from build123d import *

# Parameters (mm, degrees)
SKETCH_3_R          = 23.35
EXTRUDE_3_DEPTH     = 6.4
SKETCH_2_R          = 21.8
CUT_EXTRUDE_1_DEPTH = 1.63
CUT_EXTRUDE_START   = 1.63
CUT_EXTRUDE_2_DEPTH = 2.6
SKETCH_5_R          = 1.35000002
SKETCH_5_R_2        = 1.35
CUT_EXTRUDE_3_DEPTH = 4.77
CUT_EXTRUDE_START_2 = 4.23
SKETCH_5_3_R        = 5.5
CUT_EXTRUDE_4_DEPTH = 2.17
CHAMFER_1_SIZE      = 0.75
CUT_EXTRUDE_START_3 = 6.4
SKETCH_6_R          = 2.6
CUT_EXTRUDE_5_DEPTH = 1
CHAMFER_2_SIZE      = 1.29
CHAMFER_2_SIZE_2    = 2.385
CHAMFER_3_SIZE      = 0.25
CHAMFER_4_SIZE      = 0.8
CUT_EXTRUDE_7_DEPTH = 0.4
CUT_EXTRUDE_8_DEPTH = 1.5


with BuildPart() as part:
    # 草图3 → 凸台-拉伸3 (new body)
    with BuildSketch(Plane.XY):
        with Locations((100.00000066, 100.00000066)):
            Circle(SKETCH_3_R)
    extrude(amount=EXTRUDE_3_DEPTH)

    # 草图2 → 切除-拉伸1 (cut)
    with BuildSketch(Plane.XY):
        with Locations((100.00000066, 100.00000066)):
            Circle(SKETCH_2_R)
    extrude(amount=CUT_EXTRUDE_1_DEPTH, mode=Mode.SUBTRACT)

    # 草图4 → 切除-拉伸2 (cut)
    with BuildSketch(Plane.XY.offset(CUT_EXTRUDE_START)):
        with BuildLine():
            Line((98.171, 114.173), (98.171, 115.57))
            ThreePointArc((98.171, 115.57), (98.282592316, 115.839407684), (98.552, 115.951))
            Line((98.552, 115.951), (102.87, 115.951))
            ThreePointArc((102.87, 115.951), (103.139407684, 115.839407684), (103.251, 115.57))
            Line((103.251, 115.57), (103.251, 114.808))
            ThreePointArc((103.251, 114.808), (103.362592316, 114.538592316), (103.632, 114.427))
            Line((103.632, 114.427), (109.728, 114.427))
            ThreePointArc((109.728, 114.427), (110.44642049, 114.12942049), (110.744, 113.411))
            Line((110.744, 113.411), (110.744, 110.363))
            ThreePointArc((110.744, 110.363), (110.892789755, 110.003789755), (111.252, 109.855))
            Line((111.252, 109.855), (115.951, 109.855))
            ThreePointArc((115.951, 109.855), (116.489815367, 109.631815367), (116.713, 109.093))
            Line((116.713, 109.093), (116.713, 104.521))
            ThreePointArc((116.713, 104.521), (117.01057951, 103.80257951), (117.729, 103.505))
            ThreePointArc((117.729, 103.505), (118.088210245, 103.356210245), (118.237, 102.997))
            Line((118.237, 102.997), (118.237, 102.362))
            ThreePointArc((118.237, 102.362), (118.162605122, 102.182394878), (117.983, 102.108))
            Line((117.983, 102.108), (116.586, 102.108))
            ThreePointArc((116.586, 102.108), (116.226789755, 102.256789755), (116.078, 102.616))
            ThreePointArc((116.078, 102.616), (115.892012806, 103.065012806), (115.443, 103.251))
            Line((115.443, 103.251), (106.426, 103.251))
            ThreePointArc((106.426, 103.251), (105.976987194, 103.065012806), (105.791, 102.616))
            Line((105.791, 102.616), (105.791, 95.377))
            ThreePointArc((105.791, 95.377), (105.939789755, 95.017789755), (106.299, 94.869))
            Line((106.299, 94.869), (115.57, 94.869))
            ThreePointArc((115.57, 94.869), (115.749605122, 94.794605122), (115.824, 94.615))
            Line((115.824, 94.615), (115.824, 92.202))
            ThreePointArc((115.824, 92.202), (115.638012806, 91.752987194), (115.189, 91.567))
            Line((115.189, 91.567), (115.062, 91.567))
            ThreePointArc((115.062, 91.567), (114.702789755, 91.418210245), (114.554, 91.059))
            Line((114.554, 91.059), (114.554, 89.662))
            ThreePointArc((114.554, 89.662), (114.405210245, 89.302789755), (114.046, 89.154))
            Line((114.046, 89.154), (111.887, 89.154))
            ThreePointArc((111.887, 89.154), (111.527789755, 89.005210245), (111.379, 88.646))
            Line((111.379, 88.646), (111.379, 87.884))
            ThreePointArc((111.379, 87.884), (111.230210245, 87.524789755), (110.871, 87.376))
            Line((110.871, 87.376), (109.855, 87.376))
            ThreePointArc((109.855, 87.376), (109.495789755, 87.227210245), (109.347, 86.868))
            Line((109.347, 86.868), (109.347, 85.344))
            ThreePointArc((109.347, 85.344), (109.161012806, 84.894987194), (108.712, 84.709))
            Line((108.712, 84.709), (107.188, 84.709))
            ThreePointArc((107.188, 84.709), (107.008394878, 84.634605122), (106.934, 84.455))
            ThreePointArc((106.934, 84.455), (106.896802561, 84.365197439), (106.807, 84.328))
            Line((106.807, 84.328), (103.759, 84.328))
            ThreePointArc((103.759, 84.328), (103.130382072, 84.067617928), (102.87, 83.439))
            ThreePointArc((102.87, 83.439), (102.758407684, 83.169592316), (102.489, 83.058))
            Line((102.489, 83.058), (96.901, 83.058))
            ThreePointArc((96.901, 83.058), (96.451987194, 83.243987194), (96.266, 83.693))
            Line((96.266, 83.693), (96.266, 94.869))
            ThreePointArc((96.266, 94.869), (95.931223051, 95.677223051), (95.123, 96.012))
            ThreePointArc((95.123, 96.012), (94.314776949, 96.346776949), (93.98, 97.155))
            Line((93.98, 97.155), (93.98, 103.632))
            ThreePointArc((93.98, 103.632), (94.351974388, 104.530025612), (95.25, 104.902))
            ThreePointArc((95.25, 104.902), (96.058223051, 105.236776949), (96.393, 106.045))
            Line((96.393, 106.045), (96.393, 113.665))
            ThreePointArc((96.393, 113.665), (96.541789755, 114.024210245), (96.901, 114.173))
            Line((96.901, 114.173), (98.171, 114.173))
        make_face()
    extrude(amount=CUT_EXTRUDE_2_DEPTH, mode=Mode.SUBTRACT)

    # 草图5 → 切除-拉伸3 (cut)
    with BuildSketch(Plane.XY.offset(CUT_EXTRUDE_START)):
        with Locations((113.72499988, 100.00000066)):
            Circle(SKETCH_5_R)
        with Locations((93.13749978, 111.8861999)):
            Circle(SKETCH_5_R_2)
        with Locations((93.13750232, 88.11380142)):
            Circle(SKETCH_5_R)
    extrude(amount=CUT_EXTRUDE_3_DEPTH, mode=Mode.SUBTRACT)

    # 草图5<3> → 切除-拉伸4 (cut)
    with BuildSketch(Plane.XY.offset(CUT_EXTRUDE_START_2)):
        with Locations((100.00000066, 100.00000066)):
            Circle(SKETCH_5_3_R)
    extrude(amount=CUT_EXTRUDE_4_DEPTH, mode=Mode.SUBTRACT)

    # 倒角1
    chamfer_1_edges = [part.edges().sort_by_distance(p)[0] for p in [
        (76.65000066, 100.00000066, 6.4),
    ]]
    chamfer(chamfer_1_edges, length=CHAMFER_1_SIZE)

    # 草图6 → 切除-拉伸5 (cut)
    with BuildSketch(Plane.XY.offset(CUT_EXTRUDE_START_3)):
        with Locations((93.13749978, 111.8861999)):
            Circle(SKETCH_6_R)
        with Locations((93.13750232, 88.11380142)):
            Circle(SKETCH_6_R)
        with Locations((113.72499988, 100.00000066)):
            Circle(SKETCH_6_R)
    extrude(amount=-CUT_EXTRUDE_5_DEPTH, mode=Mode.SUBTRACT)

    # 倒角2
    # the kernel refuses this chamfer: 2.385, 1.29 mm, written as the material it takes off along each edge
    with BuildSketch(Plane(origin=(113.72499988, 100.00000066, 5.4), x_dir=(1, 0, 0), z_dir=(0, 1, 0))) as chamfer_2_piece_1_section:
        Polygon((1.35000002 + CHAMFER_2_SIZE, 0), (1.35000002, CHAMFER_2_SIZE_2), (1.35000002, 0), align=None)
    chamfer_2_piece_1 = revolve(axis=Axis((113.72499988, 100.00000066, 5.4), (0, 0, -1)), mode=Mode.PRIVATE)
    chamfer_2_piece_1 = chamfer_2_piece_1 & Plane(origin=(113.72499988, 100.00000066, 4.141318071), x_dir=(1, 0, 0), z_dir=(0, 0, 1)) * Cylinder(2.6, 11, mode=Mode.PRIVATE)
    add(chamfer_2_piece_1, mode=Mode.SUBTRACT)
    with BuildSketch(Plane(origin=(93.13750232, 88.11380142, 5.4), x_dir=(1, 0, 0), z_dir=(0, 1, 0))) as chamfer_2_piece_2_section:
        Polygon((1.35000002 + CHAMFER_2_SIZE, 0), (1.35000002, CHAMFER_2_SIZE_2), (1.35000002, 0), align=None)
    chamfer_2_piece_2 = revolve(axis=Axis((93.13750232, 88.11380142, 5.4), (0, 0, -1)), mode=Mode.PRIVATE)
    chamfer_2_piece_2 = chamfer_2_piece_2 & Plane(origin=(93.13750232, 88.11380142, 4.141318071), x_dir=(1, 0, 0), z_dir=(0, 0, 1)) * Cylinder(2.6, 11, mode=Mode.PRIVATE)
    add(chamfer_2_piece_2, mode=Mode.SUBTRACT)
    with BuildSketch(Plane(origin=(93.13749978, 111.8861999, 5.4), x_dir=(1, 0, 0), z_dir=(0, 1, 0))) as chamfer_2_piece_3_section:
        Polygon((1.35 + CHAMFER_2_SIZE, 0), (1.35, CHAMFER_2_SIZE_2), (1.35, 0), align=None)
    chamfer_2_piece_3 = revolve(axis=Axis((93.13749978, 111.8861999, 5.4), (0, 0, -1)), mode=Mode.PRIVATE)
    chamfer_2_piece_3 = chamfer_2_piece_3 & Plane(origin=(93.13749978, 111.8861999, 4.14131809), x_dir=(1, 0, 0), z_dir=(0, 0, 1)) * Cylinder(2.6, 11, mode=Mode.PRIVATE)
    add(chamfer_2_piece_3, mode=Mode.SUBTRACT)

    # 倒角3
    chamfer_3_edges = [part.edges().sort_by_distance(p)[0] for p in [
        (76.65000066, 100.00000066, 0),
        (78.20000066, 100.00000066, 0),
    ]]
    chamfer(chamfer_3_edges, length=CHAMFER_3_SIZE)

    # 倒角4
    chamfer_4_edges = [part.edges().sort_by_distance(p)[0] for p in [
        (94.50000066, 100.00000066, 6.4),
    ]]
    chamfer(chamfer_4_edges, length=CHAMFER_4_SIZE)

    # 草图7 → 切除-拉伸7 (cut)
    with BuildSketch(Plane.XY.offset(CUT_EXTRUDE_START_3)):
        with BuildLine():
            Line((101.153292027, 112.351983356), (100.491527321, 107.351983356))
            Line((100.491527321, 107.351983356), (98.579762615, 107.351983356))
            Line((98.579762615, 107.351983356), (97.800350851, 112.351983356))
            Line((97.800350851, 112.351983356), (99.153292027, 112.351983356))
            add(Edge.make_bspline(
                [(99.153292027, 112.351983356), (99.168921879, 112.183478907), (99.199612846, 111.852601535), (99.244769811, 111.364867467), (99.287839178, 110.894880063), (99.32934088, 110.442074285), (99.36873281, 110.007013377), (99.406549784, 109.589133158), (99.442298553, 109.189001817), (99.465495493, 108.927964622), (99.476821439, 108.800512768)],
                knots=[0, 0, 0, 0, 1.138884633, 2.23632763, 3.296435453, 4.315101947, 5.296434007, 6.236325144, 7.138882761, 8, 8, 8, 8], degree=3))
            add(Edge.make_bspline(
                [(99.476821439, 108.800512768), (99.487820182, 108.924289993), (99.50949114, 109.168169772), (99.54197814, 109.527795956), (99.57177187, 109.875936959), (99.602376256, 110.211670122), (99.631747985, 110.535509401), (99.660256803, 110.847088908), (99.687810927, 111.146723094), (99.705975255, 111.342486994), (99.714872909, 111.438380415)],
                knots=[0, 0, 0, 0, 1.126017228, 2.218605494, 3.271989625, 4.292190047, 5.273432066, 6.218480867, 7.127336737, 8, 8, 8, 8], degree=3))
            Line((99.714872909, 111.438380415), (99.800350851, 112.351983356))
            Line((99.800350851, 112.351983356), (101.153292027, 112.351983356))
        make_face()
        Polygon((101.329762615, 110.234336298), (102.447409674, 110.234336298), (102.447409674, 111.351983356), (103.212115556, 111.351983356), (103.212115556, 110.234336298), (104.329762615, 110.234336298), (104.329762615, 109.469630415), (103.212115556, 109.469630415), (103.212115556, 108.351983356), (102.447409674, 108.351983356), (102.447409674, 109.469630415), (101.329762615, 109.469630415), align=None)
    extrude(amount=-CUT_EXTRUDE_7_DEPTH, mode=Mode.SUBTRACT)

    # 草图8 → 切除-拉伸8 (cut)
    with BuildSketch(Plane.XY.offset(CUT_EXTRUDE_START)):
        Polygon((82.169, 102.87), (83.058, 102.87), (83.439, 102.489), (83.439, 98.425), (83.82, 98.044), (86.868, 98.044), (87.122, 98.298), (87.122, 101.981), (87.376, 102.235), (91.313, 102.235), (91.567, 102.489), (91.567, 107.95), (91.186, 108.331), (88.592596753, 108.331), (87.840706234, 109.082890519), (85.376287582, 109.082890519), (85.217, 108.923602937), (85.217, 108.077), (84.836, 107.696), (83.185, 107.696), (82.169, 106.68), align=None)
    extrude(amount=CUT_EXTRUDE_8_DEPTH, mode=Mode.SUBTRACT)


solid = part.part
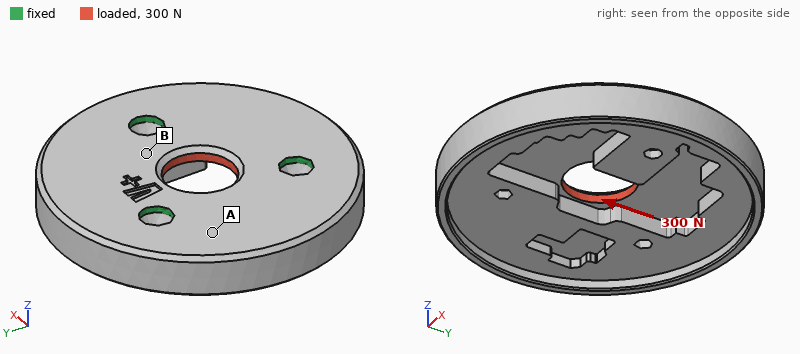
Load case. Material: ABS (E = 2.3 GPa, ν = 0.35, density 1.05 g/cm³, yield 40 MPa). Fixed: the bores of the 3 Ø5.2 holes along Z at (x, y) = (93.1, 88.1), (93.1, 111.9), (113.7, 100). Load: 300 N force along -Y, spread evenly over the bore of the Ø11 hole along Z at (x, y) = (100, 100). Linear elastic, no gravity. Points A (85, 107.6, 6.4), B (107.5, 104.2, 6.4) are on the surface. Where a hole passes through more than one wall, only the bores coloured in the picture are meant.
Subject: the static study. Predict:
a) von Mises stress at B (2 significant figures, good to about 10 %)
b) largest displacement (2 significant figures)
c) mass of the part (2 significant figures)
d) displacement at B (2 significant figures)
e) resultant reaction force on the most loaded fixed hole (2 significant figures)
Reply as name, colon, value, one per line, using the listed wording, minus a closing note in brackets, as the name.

von Mises stress at B: 2.4 MPa
largest displacement: 30 µm
mass of the part: 7.0 g
displacement at B: 13 µm
resultant reaction force on the most loaded fixed hole: 100 N
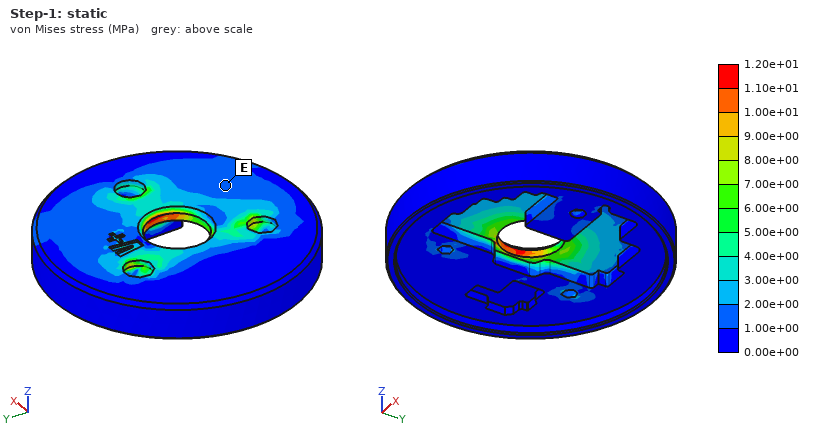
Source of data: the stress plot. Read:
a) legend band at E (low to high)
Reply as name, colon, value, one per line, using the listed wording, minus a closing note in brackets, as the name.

legend band at E: 1.00e+00 to 2.00e+00 MPa
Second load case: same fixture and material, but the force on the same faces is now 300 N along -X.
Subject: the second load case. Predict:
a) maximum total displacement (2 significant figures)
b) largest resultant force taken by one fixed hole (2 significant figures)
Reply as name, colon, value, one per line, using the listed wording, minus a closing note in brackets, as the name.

maximum total displacement: 23 µm
largest resultant force taken by one fixed hole: 100 N
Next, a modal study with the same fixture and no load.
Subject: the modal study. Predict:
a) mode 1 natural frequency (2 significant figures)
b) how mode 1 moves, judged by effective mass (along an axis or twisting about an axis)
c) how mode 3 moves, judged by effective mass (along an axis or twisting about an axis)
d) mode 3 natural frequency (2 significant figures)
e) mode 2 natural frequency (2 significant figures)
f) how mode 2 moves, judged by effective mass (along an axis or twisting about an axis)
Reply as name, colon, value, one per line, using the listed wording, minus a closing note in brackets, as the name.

mode 1 natural frequency: 2700 Hz
how mode 1 moves, judged by effective mass: twisting about X
how mode 3 moves, judged by effective mass: along Z
mode 3 natural frequency: 4200 Hz
mode 2 natural frequency: 3000 Hz
how mode 2 moves, judged by effective mass: twisting about Y
